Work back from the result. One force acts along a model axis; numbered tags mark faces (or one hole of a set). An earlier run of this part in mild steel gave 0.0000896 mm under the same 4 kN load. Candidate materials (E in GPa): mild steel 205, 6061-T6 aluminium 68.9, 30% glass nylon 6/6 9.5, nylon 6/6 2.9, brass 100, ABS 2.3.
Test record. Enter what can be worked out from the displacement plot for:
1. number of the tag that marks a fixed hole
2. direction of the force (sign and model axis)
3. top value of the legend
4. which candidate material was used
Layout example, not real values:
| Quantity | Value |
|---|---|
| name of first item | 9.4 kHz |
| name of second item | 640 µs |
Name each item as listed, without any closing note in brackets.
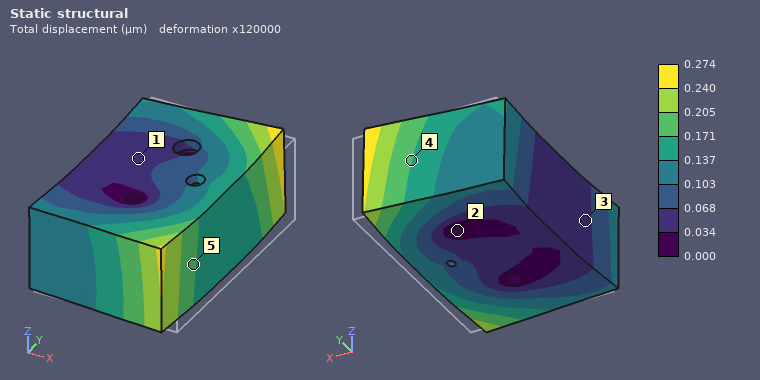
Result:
| Quantity | Value |
|---|---|
| number of the tag that marks a fixed hole | 2 |
| direction of the force | -X |
| top value of the legend | 0.274 µm |
| which candidate material was used | 6061-T6 aluminium |
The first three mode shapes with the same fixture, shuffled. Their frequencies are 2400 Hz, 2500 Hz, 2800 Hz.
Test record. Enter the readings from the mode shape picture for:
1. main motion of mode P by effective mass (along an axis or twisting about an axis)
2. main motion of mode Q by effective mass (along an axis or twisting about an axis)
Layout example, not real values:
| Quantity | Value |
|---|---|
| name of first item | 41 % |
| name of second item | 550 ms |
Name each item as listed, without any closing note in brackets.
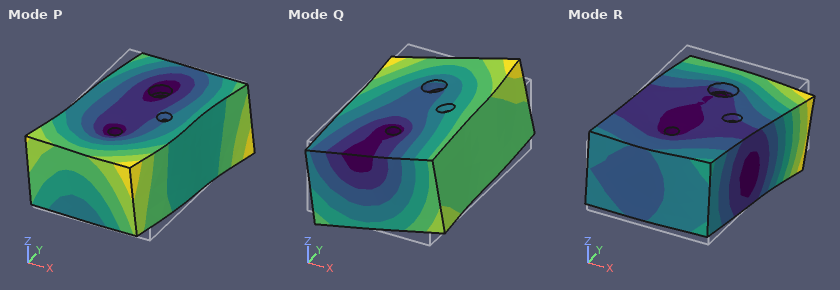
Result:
| Quantity | Value |
|---|---|
| main motion of mode P by effective mass | twisting about Z |
| main motion of mode Q by effective mass | twisting about Y |
